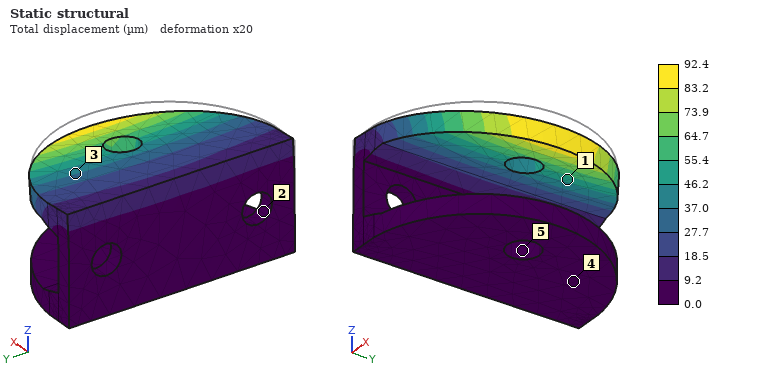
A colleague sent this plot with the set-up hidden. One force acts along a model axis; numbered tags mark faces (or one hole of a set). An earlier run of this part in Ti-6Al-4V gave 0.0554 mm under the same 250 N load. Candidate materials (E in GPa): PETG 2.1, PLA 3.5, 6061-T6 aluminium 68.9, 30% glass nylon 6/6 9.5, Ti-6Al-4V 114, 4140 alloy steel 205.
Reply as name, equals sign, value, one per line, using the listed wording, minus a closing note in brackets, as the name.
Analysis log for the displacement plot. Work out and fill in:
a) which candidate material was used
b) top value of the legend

which candidate material was used = 6061-T6 aluminium
top value of the legend = 92.4 µm
